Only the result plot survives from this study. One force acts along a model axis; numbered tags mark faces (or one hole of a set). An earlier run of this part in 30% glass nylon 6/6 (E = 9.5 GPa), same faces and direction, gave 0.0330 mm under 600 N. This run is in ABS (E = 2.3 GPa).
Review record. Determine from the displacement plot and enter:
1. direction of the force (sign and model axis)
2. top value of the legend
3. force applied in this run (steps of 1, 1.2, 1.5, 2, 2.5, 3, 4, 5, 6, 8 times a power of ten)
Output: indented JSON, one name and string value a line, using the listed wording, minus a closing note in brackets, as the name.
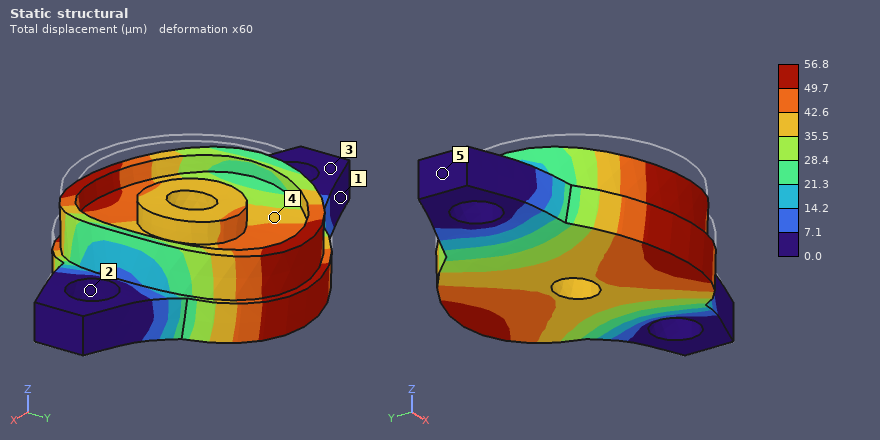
{
  "direction of the force": "-Z",
  "top value of the legend": "56.8 µm",
  "force applied in this run": "250 N"
}
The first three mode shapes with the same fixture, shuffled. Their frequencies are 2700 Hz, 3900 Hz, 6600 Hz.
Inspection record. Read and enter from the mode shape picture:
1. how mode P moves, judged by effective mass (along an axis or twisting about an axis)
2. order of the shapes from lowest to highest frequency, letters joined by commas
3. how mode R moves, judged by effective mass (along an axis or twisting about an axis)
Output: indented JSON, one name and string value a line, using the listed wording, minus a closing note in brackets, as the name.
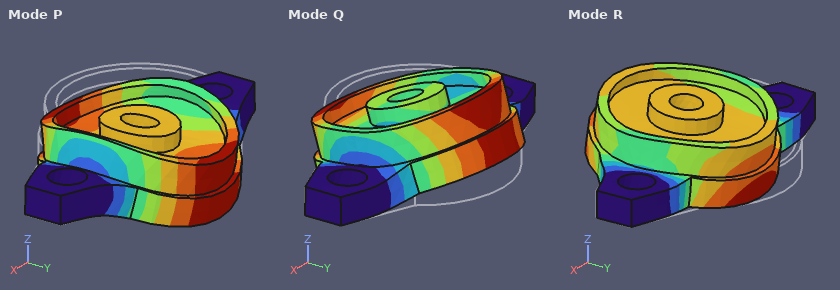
{
  "how mode P moves, judged by effective mass": "along Z",
  "order of the shapes from lowest to highest frequency, letters joined by commas": "Q, P, R",
  "how mode R moves, judged by effective mass": "along Y"
}
